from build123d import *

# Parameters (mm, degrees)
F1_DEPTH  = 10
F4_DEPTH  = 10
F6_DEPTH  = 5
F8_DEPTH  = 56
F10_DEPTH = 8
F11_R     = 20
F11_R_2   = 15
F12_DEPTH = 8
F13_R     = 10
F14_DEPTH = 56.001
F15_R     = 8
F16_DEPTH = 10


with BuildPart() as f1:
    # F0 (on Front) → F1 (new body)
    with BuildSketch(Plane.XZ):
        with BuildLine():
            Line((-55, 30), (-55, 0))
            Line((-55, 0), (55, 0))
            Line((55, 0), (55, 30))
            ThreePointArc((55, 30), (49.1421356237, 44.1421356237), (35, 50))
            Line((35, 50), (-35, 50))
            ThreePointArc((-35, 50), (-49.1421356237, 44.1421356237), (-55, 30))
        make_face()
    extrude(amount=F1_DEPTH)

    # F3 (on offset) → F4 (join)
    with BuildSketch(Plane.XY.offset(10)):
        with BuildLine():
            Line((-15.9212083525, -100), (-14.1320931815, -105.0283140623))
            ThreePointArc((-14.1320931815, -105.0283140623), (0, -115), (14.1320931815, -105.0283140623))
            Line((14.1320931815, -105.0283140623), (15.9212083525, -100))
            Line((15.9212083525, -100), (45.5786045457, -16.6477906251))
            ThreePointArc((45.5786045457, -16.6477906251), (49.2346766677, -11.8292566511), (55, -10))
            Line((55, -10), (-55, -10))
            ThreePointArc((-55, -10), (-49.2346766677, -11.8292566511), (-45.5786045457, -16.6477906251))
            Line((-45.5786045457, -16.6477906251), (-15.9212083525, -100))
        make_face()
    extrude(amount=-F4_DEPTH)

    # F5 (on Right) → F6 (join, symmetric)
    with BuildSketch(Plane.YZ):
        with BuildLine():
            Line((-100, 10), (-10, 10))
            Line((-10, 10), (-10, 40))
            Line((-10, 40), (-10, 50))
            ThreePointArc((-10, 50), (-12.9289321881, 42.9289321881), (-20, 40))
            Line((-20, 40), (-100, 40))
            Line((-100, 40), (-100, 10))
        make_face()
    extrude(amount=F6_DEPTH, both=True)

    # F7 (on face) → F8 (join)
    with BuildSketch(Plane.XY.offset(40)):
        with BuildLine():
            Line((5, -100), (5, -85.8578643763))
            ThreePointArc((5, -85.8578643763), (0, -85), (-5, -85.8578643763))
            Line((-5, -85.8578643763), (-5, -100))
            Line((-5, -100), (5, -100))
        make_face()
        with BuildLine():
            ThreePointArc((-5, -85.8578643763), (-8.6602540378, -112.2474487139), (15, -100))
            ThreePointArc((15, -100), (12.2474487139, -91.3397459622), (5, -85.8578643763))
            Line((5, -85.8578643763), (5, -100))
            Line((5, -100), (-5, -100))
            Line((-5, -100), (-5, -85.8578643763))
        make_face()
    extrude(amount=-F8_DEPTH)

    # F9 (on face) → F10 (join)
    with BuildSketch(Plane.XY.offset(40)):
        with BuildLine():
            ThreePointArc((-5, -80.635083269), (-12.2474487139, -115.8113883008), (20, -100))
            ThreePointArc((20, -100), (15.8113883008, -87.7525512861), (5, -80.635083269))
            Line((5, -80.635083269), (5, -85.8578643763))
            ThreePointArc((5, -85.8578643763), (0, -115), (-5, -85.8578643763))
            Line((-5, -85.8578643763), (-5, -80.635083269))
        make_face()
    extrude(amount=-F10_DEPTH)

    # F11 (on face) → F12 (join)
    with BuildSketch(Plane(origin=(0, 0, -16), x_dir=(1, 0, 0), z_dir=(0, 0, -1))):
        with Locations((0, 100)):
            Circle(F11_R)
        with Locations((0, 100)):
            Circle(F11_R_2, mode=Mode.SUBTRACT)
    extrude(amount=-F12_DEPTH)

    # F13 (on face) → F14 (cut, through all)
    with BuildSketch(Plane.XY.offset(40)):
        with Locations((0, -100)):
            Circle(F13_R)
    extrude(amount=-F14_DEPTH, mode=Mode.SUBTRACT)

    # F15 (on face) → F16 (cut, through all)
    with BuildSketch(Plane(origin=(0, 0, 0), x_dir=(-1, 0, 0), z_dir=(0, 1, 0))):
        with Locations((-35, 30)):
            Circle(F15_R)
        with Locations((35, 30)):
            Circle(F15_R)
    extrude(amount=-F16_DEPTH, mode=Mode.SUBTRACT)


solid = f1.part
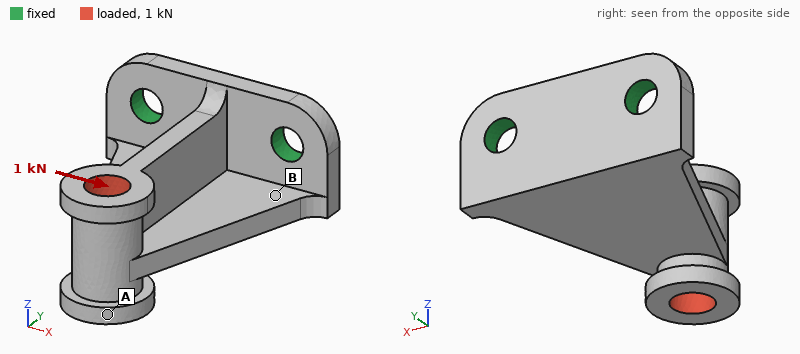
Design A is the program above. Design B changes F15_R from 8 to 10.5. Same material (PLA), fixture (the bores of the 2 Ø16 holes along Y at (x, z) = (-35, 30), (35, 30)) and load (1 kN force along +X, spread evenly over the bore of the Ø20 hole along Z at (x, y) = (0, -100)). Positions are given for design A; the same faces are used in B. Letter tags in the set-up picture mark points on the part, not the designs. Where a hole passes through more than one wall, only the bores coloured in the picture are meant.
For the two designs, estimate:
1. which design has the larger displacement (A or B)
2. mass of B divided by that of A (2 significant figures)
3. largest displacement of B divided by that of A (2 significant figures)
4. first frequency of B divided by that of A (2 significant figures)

A
0.98
0.88
1.1
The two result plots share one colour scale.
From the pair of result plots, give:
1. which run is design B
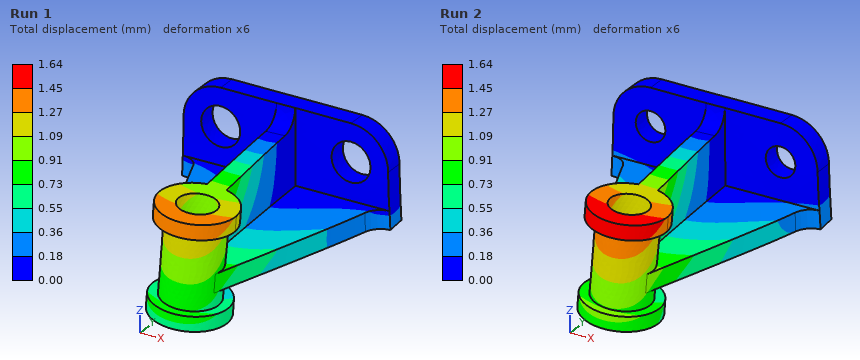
Run 1
